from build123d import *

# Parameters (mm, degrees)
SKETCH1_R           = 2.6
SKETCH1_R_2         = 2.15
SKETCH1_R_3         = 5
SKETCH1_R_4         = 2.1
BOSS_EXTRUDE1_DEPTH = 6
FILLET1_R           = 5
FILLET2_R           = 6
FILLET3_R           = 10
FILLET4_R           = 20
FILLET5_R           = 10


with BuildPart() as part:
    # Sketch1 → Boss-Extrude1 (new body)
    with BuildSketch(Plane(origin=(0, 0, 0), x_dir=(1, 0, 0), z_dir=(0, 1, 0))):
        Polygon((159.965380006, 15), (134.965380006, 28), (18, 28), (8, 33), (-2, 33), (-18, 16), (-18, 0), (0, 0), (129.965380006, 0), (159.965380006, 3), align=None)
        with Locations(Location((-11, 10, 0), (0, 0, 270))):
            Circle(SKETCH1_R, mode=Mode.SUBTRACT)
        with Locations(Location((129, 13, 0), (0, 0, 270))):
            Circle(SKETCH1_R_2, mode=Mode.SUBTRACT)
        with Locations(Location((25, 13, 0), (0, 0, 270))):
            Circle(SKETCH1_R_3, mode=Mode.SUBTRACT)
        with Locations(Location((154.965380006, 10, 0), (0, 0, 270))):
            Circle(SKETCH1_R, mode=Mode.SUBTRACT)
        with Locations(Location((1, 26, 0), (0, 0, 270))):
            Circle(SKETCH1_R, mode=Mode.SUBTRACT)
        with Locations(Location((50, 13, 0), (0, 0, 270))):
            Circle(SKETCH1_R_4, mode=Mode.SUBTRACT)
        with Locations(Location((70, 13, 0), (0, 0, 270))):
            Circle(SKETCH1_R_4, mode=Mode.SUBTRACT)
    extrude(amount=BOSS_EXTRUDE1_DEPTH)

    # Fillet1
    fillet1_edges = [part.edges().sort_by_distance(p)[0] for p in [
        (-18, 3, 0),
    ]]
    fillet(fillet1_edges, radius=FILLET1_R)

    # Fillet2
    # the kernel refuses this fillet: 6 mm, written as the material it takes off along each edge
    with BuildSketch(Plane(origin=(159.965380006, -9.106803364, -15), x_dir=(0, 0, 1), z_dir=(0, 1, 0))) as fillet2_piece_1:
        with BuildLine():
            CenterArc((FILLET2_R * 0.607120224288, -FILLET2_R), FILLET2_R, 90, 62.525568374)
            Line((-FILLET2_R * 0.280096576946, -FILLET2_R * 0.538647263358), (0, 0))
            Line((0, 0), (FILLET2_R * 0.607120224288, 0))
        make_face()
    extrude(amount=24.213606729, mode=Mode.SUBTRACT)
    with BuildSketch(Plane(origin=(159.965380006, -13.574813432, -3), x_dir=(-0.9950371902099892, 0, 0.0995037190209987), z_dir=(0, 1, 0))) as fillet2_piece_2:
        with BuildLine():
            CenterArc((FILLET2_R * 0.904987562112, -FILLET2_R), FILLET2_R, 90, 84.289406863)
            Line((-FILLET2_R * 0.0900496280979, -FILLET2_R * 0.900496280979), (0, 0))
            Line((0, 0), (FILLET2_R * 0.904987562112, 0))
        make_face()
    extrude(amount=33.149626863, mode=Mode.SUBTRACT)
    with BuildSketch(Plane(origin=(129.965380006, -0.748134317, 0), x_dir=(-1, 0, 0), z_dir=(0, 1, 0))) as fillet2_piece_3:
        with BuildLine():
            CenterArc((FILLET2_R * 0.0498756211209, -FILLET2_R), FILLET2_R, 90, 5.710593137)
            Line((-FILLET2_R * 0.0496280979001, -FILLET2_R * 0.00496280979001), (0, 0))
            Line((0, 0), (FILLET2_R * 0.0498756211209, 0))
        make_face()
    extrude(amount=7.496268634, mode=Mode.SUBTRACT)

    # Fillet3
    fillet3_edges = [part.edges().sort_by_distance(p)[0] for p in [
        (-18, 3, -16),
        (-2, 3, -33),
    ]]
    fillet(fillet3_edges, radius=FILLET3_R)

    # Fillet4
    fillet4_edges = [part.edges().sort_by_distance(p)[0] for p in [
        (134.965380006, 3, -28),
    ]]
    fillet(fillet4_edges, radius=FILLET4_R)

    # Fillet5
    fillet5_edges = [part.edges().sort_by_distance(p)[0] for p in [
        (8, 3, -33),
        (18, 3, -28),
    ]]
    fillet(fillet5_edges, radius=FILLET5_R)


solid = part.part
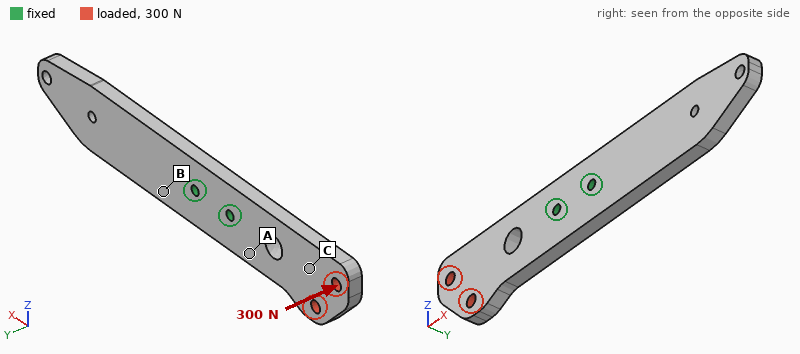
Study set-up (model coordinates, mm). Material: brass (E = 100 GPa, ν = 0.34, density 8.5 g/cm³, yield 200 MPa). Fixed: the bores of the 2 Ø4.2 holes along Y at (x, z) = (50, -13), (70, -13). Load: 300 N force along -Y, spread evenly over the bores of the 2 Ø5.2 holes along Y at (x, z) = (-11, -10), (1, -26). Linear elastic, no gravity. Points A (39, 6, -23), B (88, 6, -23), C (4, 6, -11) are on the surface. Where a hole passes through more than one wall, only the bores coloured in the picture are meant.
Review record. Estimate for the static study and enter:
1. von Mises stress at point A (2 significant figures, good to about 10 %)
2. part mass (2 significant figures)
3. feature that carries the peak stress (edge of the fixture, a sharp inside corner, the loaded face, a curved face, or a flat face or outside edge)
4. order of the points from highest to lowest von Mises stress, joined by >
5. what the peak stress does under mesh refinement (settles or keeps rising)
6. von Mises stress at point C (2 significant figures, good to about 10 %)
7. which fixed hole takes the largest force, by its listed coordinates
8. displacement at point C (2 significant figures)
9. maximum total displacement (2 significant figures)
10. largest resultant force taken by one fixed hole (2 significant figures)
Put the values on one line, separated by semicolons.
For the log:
77 MPa; 230 g; edge of the fixture; A > C > B; keeps rising; 18 MPa; (50, -13); 0.28 mm; 0.51 mm; 610 N
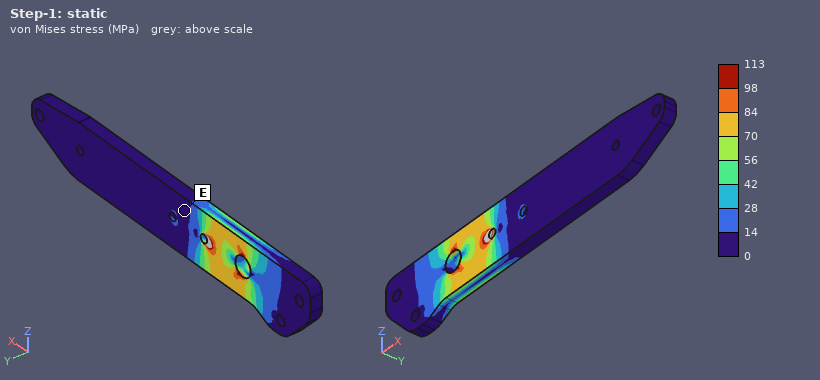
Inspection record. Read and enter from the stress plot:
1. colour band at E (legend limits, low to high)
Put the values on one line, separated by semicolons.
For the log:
0 to 14 MPa
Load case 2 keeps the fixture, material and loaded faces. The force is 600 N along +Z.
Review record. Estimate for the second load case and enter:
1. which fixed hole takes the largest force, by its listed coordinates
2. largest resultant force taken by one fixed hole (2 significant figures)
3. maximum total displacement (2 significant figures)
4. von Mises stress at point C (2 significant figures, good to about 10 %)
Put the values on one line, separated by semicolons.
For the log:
(50, -13); 1.9 kN; 82 µm; 8.0 MPa
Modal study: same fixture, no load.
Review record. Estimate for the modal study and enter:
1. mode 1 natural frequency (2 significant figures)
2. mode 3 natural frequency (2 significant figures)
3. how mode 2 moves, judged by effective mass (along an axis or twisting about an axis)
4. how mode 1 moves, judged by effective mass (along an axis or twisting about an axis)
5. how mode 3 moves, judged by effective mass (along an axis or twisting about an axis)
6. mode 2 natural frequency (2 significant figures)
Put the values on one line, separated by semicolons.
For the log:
480 Hz; 1600 Hz; along Y; along Y; along Z; 720 Hz
